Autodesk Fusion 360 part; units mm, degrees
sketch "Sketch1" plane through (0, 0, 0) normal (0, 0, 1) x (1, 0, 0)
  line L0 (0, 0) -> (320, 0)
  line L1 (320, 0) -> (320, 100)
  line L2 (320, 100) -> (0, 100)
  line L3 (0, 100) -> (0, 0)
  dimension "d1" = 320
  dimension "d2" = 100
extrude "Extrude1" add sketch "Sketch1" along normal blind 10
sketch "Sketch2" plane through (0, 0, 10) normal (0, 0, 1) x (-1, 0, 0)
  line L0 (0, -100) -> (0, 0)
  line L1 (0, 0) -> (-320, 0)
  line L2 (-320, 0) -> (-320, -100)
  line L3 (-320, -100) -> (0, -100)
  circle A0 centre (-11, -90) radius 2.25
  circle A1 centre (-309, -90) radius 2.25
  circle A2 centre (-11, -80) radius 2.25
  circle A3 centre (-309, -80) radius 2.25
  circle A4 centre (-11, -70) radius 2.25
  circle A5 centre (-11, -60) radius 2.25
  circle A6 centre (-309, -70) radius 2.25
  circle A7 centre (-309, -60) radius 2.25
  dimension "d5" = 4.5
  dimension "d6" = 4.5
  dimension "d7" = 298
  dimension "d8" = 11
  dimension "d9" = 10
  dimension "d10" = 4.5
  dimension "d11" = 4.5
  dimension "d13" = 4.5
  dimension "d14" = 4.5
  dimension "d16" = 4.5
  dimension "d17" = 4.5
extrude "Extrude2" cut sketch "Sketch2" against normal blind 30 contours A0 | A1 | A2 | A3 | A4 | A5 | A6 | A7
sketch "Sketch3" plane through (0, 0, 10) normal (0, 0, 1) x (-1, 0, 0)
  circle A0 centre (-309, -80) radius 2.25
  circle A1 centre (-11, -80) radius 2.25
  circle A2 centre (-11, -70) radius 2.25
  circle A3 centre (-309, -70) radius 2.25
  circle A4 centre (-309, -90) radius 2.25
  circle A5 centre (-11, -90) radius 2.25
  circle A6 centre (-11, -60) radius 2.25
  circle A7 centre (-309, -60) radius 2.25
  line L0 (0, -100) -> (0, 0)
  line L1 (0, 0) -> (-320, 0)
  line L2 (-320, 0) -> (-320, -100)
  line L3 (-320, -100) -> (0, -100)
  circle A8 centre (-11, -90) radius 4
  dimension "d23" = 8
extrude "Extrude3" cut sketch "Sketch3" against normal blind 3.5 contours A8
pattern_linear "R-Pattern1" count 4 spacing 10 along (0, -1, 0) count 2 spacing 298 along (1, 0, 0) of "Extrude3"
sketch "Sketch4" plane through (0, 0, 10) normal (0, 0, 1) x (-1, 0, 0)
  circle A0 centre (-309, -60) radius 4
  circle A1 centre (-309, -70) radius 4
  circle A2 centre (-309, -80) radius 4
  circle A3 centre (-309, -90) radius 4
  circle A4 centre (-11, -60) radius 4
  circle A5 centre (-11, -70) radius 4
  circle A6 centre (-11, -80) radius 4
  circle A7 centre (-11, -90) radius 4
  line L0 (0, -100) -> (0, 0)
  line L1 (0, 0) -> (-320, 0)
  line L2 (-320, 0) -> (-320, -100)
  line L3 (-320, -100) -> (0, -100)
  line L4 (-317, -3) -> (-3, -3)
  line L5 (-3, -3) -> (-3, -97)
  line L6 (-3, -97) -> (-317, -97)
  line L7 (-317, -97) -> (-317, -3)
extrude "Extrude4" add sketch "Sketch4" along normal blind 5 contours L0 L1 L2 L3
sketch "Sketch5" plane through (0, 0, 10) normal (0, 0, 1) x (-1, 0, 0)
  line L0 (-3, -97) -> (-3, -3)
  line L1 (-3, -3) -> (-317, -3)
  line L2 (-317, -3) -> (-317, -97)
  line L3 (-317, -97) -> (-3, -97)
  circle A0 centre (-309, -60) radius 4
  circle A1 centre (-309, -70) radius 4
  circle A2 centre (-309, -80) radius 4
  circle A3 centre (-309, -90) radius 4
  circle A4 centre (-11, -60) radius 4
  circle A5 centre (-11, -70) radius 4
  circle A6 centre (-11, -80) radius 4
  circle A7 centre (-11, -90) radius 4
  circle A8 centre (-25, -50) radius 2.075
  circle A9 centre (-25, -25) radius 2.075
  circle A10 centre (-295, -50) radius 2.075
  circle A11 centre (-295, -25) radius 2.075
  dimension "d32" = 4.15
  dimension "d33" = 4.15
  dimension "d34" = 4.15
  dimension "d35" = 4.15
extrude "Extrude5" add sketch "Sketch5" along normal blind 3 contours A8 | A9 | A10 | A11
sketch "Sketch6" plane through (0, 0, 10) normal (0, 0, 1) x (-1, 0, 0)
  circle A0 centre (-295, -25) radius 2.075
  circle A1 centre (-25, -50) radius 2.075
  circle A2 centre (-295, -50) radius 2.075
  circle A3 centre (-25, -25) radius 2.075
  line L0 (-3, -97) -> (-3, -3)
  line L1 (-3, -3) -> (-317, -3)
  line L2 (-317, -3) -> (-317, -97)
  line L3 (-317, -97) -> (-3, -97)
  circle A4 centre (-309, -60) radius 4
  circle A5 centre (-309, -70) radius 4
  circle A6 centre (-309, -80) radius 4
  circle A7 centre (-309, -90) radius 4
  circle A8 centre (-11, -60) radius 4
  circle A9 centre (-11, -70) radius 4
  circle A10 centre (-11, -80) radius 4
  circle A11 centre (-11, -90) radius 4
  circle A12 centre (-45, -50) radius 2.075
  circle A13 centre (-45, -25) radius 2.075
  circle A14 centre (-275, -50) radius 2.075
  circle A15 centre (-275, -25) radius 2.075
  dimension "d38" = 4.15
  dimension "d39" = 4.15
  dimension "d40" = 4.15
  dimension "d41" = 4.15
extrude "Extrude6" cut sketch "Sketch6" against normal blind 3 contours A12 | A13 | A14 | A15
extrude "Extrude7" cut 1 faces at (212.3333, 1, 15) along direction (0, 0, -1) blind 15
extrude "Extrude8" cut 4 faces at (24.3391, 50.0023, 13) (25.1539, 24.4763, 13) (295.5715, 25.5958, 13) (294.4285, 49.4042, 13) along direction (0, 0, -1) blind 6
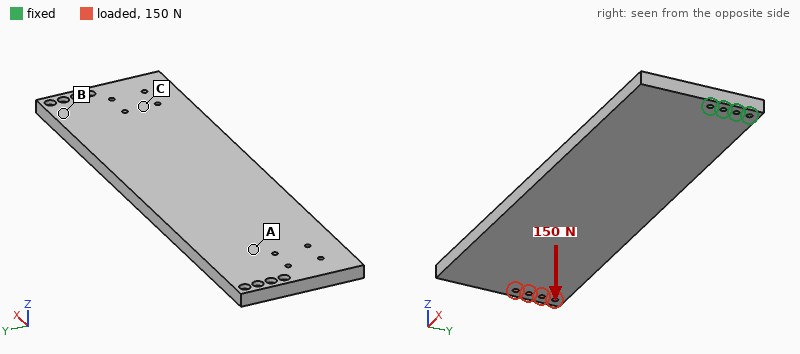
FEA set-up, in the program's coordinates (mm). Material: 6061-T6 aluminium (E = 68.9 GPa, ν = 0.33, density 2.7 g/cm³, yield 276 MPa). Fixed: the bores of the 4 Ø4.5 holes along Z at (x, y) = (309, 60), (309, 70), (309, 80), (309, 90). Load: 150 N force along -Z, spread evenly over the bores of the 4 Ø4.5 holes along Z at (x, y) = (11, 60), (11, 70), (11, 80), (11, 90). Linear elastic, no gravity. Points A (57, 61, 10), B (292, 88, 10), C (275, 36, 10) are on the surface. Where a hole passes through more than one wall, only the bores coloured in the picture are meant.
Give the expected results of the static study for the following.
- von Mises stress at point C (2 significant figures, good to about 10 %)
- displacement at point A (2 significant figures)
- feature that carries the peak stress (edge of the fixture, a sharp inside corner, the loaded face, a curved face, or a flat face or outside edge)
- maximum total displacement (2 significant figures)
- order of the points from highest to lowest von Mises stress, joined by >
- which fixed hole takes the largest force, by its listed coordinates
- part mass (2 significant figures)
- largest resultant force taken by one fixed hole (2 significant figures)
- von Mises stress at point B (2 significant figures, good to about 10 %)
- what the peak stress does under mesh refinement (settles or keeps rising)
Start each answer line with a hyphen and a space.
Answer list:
- 23 MPa
- 2.4 mm
- edge of the fixture
- 3.2 mm
- B > C > A
- (309, 70)
- 790 g
- 400 N
- 40 MPa
- keeps rising
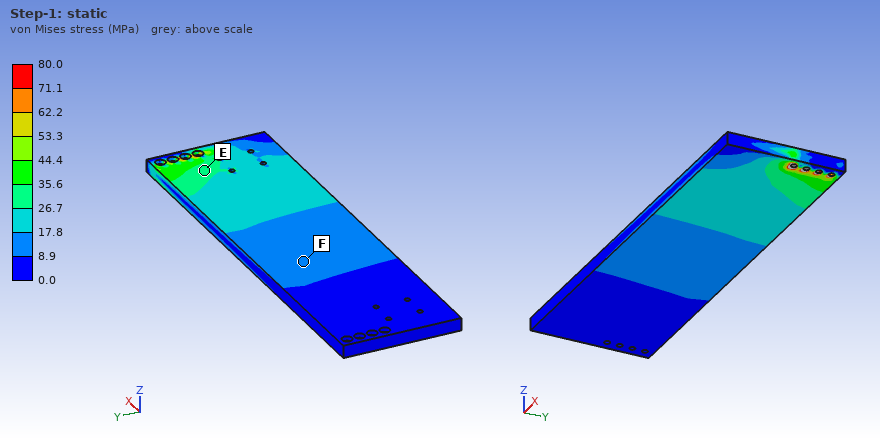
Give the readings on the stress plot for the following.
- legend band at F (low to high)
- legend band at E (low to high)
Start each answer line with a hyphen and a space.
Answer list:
- 8.9 to 17.8 MPa
- 26.7 to 35.6 MPa
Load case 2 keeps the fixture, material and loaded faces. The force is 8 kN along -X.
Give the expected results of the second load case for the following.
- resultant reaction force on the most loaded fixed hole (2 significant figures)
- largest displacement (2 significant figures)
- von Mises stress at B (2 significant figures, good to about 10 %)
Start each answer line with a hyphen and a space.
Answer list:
- 2.4 kN
- 1.3 mm
- 8.8 MPa
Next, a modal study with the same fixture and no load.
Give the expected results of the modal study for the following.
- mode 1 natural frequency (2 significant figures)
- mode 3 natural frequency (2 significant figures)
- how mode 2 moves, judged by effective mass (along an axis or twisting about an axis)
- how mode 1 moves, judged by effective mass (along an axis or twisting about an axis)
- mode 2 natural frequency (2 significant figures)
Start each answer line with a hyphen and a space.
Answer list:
- 76 Hz
- 460 Hz
- along Y
- along Z
- 400 Hz
